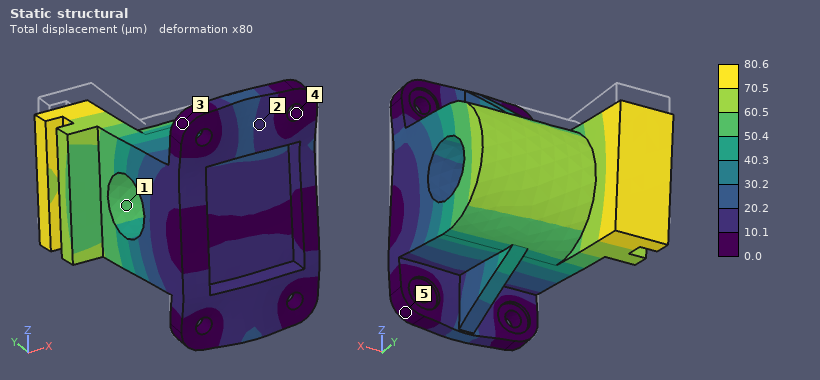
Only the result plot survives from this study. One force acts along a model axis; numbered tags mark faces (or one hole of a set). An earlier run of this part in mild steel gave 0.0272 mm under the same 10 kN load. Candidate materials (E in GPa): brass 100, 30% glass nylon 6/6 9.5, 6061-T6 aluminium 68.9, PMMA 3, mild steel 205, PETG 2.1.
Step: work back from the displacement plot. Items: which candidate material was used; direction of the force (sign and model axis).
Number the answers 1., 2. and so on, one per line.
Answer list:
1. 6061-T6 aluminium
2. -Z
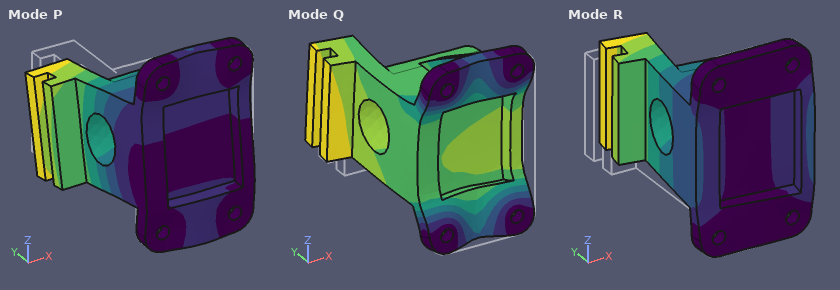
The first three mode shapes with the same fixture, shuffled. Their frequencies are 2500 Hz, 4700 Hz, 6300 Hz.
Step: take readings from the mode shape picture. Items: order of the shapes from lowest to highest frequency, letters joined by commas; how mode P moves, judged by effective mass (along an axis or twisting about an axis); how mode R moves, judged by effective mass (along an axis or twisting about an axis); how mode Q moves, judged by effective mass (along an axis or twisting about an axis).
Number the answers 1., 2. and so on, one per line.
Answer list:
1. R, P, Q
2. along Z
3. along X
4. along Y
